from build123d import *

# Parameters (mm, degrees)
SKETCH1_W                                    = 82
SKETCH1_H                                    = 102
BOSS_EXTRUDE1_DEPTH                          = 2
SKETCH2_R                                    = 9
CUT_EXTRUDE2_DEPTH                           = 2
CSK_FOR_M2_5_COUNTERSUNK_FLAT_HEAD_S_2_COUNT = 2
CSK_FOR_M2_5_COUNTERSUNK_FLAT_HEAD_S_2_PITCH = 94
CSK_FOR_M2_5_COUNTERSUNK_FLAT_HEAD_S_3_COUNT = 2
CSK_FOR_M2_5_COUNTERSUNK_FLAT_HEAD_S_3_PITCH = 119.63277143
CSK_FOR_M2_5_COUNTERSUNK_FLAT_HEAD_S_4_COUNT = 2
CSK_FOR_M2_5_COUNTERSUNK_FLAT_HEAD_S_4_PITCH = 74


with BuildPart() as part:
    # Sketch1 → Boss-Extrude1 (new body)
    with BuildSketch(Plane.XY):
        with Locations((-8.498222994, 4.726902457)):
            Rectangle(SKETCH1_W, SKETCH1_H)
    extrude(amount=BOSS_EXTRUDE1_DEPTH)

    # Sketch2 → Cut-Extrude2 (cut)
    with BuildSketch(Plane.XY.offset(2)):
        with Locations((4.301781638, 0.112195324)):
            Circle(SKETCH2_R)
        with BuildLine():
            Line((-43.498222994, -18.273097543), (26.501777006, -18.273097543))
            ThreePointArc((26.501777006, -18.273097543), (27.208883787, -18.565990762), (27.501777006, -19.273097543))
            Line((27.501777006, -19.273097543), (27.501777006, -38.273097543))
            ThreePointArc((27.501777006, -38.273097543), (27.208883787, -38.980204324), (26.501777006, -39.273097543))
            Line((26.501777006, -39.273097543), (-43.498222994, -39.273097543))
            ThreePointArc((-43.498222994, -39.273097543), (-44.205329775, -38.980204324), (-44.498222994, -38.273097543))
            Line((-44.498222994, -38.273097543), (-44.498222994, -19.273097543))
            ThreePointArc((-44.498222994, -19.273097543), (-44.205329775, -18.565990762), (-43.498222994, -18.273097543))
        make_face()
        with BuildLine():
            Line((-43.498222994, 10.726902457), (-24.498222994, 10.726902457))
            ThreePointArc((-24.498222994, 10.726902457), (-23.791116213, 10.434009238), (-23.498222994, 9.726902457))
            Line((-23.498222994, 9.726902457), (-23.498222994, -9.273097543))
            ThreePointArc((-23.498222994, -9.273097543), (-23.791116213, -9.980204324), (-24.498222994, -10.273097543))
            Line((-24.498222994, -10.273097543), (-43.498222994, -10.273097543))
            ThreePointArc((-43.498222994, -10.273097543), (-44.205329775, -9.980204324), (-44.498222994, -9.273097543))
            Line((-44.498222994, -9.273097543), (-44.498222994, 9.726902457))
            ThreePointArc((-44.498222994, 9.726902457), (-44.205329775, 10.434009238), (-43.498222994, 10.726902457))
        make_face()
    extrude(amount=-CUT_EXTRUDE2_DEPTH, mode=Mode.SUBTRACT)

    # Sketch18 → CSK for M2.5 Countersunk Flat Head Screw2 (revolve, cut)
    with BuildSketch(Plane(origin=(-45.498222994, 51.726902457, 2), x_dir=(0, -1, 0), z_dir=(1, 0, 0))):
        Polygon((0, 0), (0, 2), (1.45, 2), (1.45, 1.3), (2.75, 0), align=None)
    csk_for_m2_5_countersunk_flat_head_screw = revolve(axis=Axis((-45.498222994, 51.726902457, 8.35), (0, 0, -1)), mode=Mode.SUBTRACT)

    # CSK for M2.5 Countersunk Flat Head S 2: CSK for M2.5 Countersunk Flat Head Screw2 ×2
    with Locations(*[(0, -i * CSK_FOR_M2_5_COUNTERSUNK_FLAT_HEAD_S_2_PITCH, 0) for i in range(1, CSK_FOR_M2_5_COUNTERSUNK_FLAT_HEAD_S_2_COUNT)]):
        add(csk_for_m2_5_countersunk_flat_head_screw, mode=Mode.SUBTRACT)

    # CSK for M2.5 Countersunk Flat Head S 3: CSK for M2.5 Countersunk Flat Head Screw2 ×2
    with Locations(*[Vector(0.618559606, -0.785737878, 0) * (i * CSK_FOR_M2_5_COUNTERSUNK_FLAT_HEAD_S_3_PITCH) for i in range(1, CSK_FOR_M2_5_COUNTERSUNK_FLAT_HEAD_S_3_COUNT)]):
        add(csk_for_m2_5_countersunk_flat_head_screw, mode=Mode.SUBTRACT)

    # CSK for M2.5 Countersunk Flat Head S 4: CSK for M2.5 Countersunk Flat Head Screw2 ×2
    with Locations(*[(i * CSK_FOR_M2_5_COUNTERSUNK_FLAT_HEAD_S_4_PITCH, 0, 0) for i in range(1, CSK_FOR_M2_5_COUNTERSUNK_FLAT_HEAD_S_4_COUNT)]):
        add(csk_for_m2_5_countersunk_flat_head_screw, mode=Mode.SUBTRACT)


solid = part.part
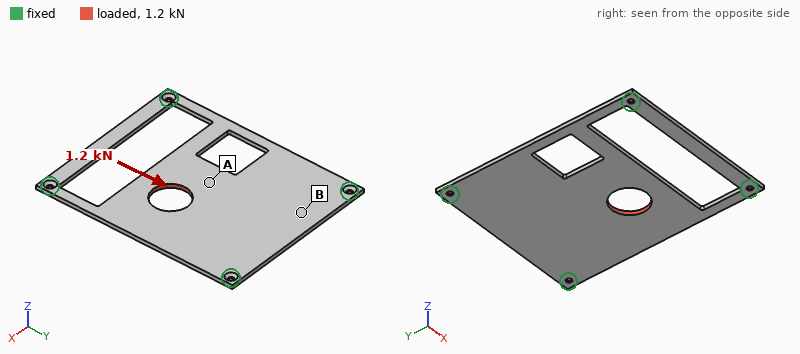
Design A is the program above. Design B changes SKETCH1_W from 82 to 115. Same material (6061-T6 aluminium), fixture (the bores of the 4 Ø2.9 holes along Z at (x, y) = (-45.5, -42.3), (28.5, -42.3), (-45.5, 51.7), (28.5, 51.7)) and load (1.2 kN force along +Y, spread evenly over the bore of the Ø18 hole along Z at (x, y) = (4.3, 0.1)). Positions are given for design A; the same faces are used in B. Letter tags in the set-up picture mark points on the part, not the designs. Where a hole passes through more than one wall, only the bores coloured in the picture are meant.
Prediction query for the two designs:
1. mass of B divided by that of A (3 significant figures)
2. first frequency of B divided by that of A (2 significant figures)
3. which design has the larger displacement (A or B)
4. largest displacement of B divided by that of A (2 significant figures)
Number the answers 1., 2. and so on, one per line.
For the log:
1. 1.55
2. 1.1
3. A
4. 0.78
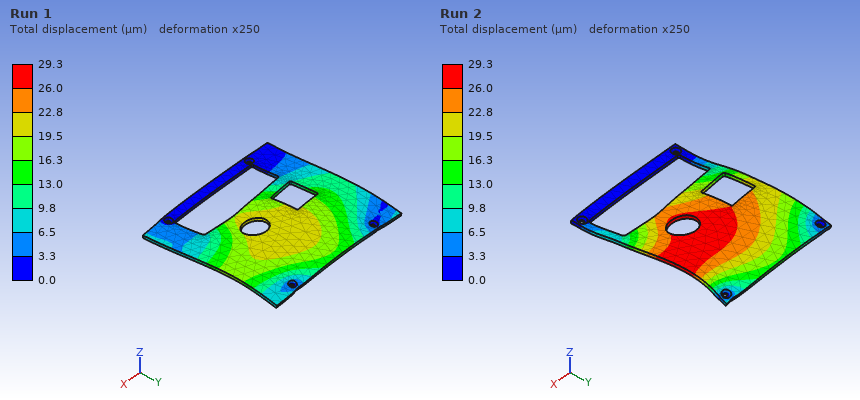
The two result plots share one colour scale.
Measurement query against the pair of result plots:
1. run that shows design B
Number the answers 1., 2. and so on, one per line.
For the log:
1. Run 1
